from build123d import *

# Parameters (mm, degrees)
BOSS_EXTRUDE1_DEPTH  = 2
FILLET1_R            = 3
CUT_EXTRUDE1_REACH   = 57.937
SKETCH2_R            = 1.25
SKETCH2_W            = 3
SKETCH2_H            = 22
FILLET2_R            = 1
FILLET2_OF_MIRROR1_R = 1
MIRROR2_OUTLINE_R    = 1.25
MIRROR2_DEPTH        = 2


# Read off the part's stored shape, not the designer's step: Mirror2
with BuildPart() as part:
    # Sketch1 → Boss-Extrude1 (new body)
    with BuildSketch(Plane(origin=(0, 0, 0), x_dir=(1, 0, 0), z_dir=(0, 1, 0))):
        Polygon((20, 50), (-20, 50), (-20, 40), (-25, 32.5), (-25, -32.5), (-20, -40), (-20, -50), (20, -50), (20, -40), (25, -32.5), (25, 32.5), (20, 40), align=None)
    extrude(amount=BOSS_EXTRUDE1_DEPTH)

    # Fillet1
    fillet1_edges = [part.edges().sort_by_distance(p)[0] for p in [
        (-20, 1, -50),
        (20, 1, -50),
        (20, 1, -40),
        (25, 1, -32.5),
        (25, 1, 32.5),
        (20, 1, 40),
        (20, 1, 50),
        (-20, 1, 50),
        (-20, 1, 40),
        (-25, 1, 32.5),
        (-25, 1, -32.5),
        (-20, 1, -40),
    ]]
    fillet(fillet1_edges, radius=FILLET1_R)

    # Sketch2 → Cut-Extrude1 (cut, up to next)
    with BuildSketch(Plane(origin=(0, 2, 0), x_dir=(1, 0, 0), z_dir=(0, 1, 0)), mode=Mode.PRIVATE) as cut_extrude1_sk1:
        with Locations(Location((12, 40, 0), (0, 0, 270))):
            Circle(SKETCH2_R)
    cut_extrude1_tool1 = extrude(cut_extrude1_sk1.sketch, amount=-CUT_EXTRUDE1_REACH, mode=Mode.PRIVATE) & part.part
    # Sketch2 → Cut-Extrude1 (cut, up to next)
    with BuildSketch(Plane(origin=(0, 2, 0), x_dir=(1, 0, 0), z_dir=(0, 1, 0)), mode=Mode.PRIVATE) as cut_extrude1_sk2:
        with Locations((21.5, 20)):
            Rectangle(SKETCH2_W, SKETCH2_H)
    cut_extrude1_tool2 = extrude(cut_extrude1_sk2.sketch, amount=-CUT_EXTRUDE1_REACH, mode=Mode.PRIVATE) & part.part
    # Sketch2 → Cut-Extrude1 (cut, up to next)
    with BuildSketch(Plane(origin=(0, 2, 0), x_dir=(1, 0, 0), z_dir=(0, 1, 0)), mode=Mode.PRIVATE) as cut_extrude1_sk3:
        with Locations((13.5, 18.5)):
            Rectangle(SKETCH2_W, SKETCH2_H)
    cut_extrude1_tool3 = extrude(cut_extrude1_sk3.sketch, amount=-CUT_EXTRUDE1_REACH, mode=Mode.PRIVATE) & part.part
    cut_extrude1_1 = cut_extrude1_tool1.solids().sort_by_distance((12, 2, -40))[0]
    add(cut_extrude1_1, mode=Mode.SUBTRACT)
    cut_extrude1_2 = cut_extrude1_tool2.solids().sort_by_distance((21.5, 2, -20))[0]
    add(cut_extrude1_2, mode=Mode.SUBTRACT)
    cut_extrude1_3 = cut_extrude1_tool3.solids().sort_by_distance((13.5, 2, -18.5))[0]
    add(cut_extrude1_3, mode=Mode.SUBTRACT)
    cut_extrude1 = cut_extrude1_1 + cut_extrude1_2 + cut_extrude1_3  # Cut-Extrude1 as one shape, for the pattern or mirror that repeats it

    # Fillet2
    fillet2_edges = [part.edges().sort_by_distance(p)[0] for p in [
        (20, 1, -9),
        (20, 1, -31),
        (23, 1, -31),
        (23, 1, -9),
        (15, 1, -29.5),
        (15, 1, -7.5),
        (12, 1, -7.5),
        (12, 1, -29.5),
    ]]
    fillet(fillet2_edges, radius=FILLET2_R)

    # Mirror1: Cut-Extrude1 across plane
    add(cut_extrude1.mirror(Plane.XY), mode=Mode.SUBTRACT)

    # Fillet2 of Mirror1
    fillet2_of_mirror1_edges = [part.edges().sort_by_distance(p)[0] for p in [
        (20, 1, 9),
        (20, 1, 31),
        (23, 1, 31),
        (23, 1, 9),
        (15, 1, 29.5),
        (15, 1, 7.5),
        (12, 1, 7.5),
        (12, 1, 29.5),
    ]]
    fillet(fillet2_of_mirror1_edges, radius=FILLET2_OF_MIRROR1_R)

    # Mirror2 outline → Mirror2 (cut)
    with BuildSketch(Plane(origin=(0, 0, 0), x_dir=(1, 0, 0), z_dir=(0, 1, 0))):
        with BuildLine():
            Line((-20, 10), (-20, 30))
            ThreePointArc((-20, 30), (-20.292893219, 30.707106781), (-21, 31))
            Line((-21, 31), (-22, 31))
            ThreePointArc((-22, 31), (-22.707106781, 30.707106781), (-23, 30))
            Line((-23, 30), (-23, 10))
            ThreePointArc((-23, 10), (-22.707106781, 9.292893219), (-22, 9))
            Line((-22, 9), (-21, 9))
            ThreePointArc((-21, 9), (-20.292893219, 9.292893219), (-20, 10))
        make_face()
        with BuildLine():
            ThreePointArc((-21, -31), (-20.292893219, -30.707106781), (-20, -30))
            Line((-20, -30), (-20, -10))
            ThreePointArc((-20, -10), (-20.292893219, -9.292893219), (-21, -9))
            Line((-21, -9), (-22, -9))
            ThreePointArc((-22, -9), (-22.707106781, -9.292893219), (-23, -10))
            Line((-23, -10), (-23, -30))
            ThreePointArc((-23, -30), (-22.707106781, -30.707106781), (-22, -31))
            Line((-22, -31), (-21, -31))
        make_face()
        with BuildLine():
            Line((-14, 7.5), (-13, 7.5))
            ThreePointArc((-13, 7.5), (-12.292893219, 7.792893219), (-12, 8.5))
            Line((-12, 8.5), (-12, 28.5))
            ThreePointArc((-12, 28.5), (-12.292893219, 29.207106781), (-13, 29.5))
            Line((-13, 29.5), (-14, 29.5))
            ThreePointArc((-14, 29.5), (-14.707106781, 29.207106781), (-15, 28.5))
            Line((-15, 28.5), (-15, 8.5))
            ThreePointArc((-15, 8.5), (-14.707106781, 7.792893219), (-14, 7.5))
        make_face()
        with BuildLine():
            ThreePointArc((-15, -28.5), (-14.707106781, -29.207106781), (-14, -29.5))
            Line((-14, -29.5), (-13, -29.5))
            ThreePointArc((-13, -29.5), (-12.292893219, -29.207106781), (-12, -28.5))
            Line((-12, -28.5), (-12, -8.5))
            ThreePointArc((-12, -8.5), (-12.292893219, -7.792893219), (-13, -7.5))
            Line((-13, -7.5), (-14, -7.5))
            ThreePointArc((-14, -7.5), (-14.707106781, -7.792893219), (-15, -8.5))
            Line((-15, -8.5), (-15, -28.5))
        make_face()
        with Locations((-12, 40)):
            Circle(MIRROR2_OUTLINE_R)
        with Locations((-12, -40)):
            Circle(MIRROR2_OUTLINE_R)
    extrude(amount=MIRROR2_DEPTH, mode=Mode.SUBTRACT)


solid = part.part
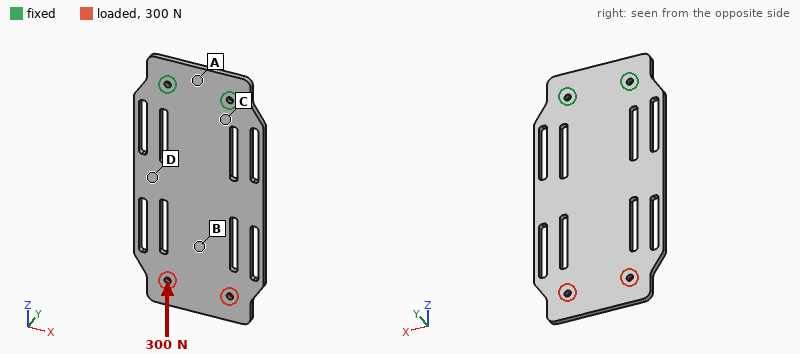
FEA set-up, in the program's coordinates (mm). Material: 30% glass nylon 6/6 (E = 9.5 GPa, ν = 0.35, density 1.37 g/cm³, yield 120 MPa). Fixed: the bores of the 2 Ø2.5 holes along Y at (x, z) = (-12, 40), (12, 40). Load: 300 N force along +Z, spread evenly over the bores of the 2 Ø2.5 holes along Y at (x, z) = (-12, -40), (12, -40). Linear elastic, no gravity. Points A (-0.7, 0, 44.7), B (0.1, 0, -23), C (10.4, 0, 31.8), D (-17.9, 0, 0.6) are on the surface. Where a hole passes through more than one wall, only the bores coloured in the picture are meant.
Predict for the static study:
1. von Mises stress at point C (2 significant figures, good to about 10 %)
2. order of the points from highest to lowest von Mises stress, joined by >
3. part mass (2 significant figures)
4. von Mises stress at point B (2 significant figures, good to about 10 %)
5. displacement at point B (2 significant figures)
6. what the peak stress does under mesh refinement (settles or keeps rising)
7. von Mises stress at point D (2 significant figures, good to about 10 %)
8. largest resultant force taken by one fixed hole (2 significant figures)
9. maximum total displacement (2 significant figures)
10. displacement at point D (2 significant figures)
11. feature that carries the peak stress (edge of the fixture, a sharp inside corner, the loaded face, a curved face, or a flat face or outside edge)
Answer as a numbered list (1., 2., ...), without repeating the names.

1. 5.6 MPa
2. C > B > D > A
3. 11 g
4. 3.6 MPa
5. 28 µm
6. keeps rising
7. 2.5 MPa
8. 150 N
9. 39 µm
10. 19 µm
11. edge of the fixture
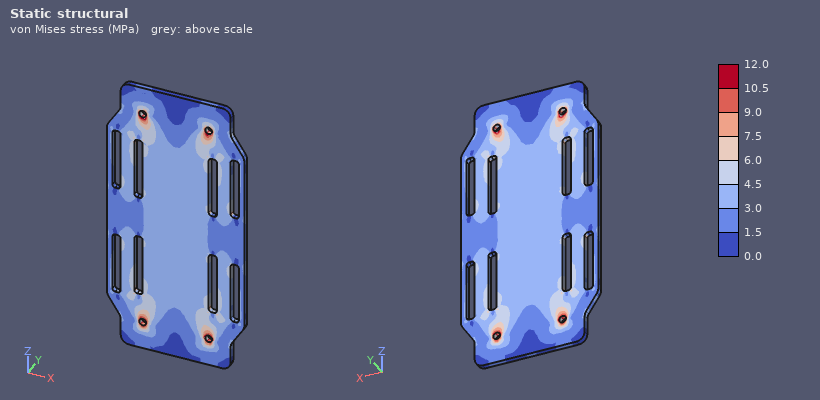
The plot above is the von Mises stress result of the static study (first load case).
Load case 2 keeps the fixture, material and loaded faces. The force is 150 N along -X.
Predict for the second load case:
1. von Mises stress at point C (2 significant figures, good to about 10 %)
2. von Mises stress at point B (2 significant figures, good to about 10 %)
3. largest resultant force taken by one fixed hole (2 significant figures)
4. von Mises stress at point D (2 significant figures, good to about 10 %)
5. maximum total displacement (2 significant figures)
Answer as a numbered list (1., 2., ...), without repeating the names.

1. 20 MPa
2. 6.6 MPa
3. 480 N
4. 6.6 MPa
5. 0.43 mm
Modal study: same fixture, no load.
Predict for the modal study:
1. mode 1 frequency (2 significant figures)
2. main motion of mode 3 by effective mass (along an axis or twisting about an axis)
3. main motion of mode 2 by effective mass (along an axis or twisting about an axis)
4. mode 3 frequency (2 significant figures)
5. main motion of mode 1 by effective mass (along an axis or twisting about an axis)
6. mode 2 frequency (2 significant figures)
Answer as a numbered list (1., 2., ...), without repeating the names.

1. 100 Hz
2. along Y
3. twisting about Z
4. 640 Hz
5. along Y
6. 420 Hz
